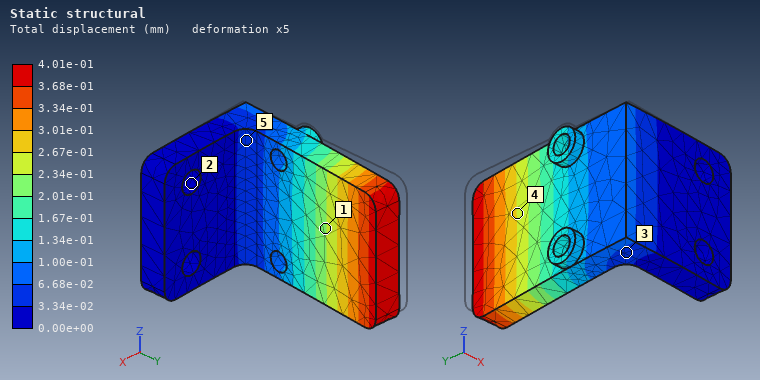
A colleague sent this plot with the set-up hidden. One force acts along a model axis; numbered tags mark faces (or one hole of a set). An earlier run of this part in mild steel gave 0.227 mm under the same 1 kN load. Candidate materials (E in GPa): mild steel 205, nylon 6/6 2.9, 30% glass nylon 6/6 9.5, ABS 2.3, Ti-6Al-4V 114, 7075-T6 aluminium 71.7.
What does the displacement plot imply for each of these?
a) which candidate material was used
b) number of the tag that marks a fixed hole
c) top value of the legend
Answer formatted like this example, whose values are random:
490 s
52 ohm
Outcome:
Ti-6Al-4V
2
4.01e-01 mm
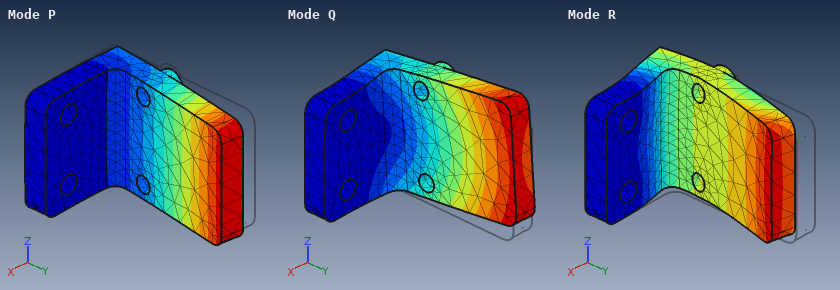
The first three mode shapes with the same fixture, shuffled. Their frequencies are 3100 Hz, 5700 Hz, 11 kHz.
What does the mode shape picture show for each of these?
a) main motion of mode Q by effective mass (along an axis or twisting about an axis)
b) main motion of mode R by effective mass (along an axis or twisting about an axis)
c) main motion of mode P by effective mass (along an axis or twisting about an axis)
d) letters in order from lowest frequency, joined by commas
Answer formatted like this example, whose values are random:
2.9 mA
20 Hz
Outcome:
along Z
along Y
along X
P, Q, R
